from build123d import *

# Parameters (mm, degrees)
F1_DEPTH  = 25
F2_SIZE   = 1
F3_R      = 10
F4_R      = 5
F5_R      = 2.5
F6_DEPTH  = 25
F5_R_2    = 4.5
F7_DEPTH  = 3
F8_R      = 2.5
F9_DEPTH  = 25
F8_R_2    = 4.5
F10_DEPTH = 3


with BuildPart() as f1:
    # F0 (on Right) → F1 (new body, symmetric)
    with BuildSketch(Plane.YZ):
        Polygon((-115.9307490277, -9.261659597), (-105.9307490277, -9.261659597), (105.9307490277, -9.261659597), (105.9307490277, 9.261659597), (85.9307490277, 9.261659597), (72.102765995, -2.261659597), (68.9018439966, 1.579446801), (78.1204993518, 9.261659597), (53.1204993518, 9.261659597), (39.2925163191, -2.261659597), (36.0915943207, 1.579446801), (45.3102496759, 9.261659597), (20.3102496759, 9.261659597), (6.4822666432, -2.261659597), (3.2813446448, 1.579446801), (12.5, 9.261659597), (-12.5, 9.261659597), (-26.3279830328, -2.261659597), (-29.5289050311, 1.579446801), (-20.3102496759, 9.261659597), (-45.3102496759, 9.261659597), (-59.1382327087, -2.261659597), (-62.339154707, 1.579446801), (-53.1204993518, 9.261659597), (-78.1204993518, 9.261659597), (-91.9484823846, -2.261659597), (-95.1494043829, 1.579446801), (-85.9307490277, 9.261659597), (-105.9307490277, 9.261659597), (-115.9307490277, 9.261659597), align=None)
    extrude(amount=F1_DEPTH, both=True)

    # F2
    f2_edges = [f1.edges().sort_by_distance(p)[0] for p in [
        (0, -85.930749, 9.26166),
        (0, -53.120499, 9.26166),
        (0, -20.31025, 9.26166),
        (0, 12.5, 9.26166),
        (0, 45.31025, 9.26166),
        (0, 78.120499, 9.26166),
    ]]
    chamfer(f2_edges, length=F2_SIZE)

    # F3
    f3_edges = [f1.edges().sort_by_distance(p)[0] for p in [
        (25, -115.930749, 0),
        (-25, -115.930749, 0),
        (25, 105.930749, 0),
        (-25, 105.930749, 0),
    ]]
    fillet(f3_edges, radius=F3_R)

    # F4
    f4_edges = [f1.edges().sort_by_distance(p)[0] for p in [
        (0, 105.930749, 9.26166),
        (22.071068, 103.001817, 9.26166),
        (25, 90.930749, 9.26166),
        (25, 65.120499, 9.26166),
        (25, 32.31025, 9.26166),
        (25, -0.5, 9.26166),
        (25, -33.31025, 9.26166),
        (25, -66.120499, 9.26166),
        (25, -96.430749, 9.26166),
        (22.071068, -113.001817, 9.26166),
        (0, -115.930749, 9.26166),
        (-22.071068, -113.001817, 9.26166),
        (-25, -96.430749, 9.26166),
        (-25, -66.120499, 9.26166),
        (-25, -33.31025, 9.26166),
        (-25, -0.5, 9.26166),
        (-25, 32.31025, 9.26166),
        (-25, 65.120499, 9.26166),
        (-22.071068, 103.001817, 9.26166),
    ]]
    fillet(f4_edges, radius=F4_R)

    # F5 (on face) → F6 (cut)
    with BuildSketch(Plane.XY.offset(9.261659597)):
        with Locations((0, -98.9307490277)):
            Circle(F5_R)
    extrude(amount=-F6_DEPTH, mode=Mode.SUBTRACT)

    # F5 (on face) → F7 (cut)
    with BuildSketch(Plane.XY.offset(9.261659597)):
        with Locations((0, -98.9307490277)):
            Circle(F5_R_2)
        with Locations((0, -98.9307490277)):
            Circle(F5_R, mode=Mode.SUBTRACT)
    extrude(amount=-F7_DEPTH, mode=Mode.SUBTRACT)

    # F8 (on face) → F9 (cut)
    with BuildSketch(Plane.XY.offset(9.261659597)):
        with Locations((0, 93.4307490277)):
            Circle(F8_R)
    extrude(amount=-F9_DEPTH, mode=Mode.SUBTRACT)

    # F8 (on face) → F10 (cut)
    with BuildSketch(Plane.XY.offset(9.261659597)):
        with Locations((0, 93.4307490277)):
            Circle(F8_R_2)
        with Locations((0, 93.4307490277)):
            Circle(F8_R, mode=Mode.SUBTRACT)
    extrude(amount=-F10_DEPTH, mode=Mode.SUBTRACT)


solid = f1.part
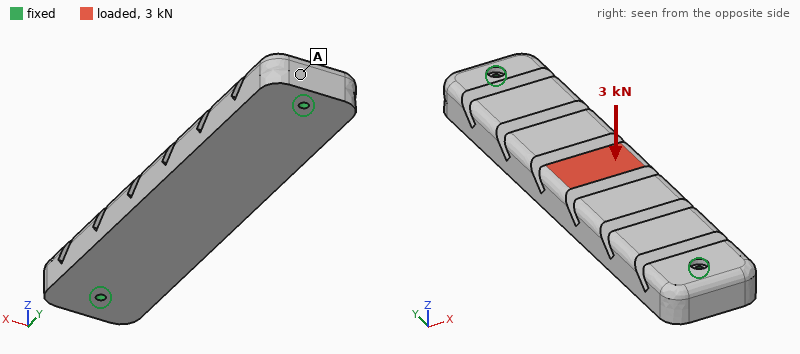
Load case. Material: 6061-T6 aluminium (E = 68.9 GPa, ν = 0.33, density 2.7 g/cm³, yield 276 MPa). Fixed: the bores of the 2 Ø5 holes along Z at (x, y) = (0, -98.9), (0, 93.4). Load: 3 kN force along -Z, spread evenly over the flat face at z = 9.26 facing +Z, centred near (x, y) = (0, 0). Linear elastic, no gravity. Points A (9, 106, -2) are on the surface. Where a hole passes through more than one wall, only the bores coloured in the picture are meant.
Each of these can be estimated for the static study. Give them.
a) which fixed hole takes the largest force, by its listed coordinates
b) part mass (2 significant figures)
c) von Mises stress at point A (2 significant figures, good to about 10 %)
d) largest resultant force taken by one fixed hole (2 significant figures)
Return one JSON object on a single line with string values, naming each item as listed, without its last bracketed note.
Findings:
{"which fixed hole takes the largest force, by its listed coordinates": "(0, 93.4)", "part mass": "480 g", "von Mises stress at point A": "17 MPa", "largest resultant force taken by one fixed hole": "1.7 kN"}
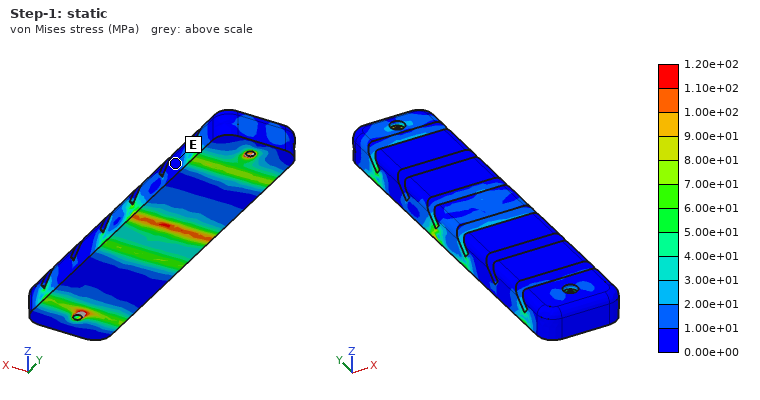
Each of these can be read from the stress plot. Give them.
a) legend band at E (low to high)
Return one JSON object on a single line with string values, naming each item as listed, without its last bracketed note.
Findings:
{"legend band at E": "0.00e+00 to 1.00e+01 MPa"}
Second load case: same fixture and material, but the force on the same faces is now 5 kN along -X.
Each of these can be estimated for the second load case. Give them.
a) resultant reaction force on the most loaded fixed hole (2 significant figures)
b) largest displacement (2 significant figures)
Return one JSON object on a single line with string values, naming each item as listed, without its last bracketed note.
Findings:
{"resultant reaction force on the most loaded fixed hole": "2.6 kN", "largest displacement": "0.16 mm"}
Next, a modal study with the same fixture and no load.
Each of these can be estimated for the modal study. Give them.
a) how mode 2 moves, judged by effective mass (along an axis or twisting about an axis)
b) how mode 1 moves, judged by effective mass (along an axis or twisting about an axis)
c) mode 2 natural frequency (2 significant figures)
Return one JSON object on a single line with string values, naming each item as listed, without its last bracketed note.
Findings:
{"how mode 2 moves, judged by effective mass": "along X", "how mode 1 moves, judged by effective mass": "along Z", "mode 2 natural frequency": "2400 Hz"}
